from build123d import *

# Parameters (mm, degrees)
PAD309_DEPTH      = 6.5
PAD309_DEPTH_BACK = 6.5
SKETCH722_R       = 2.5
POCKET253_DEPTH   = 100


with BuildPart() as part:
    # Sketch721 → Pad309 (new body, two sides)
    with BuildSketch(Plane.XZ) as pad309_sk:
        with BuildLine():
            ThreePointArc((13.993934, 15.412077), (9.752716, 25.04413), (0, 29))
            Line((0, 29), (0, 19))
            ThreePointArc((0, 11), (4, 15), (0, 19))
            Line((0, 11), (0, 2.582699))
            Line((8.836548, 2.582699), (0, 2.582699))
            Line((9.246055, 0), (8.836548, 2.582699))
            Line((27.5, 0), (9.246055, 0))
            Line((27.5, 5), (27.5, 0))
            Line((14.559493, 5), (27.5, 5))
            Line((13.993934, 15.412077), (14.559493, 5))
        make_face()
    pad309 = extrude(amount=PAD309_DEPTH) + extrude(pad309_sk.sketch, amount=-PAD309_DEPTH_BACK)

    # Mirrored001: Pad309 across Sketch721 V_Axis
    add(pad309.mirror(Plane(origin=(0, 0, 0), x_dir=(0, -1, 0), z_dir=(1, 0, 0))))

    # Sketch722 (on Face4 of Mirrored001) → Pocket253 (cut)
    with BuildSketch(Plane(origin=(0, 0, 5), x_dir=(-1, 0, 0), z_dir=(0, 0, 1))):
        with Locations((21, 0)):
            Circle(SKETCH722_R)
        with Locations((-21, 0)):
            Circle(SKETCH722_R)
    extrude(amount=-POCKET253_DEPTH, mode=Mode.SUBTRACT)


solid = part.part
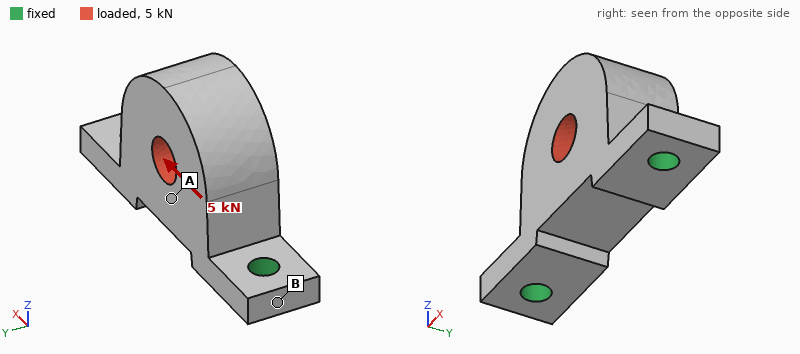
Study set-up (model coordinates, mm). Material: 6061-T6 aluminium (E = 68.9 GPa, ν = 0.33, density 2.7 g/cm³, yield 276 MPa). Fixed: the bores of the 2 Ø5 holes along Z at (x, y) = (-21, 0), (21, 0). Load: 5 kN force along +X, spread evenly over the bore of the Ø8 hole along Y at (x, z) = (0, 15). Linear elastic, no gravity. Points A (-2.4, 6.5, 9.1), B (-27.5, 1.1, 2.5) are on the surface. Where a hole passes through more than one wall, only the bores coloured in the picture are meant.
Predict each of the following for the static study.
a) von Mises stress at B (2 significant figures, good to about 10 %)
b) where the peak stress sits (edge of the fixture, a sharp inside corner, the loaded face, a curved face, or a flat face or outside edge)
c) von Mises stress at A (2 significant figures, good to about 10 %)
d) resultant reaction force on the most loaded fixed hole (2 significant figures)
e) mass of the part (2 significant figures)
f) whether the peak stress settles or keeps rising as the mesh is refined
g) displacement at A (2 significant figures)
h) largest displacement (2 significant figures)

14 MPa
edge of the fixture
32 MPa
3.1 kN
27 g
keeps rising
13 µm
37 µm
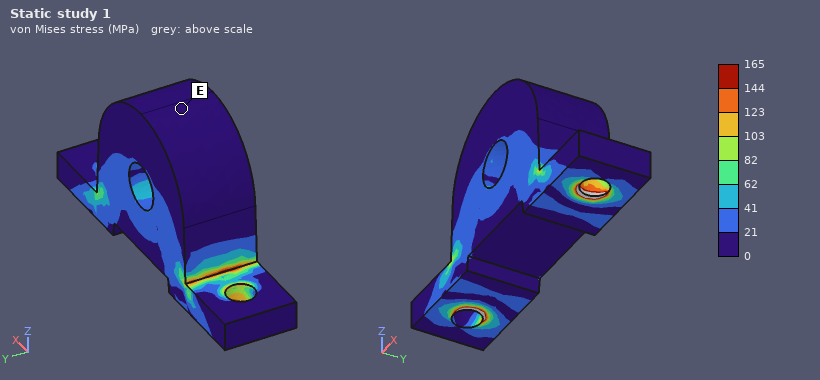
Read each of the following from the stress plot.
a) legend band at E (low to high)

0 to 21 MPa
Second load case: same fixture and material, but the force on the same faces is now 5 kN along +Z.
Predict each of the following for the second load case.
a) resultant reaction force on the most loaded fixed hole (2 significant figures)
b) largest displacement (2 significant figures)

3.1 kN
32 µm
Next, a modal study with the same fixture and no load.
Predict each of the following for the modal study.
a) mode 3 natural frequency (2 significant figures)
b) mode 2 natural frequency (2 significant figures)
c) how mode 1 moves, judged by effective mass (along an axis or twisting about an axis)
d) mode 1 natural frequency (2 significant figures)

14 kHz
14 kHz
along Y
4400 Hz
